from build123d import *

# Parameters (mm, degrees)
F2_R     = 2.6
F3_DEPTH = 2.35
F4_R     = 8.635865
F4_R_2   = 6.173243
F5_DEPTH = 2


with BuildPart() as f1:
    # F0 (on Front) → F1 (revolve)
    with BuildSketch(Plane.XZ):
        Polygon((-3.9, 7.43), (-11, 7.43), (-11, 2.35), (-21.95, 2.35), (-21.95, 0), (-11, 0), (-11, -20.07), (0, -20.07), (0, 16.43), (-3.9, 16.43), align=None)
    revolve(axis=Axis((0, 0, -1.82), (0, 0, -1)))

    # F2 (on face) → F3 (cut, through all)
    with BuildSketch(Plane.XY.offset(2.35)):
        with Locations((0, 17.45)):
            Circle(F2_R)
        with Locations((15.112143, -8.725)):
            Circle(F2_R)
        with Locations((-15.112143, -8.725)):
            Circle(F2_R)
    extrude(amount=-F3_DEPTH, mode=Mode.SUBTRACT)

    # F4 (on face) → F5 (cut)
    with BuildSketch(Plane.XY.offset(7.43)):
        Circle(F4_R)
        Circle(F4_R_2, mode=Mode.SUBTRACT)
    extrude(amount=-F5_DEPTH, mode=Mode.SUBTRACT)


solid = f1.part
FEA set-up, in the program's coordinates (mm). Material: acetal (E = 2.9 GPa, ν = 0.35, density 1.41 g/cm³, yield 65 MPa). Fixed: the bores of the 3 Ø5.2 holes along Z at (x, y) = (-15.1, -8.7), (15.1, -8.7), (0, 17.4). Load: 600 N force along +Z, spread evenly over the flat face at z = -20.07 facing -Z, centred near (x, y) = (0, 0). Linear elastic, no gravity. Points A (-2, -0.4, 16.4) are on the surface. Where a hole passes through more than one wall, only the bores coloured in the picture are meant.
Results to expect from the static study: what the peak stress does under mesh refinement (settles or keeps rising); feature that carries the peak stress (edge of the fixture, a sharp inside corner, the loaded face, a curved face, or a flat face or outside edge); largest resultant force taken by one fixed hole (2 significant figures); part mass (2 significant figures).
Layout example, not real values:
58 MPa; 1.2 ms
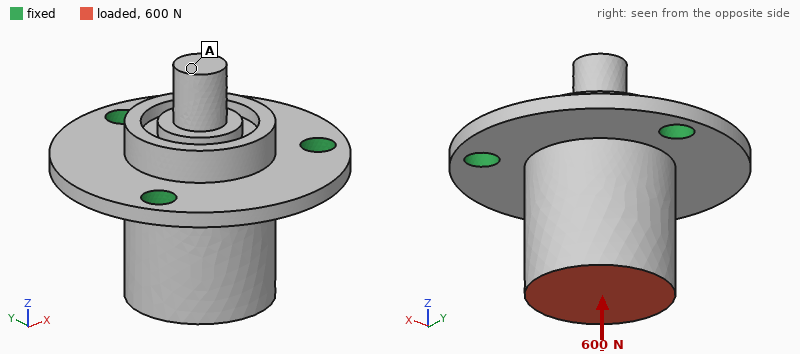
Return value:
keeps rising; edge of the fixture; 200 N; 19 g
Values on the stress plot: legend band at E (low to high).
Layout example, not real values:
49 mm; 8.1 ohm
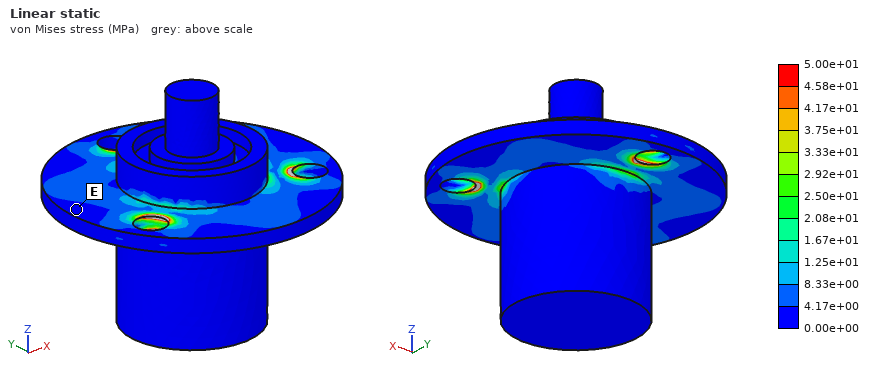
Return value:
0.00e+00 to 4.17e+00 MPa
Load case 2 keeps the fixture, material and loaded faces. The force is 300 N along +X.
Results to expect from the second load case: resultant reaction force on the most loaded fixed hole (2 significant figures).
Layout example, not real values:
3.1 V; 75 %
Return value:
270 N
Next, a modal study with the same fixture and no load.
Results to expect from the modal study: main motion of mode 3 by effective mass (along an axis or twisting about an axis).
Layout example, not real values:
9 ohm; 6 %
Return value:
along Z
